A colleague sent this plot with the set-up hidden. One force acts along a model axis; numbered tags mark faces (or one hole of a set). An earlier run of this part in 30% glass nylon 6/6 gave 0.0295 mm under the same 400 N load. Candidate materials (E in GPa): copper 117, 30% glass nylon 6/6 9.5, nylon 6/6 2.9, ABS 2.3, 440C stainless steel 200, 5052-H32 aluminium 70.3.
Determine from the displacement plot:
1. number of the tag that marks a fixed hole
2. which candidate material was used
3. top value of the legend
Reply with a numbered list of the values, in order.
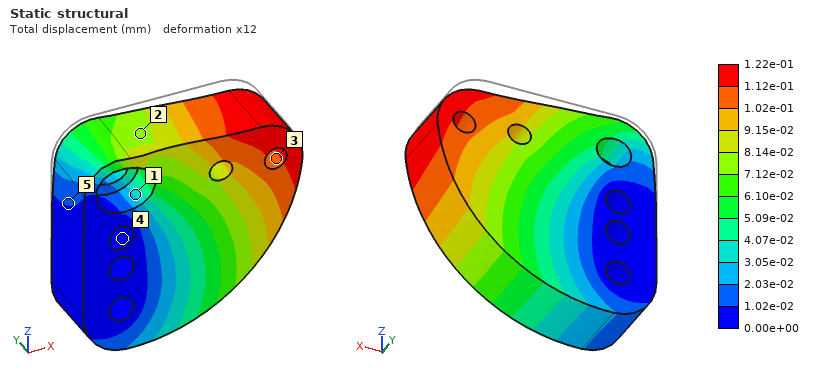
1. 4
2. ABS
3. 1.22e-01 mm
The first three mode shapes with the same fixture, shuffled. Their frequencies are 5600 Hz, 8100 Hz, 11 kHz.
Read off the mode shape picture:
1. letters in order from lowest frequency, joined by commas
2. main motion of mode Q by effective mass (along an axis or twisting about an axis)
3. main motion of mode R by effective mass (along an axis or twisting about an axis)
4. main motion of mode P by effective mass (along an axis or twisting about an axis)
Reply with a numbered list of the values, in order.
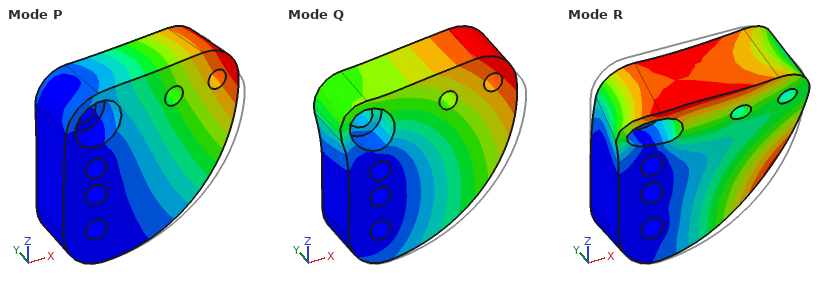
1. P, Q, R
2. along Z
3. twisting about X
4. along Y
